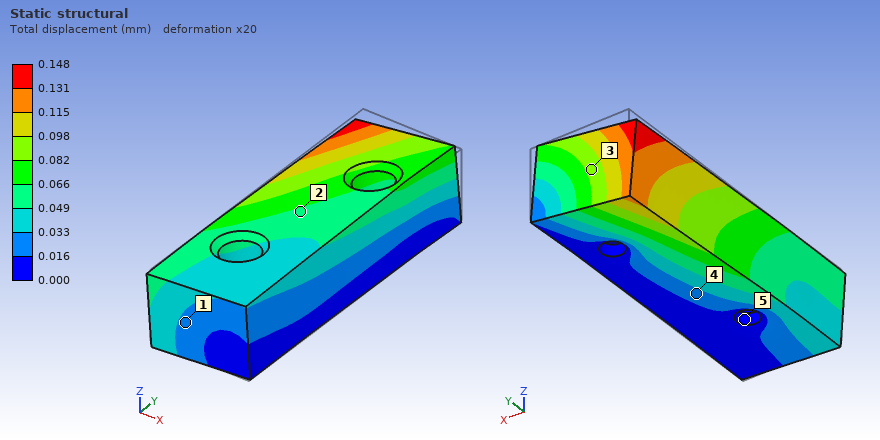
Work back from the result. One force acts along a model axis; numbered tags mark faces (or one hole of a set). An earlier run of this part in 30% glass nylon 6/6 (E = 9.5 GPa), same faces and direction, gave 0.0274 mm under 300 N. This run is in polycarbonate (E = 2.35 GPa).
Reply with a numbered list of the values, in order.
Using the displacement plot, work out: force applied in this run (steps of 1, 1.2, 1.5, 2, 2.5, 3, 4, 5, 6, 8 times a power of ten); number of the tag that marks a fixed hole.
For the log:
1. 400 N
2. 5
